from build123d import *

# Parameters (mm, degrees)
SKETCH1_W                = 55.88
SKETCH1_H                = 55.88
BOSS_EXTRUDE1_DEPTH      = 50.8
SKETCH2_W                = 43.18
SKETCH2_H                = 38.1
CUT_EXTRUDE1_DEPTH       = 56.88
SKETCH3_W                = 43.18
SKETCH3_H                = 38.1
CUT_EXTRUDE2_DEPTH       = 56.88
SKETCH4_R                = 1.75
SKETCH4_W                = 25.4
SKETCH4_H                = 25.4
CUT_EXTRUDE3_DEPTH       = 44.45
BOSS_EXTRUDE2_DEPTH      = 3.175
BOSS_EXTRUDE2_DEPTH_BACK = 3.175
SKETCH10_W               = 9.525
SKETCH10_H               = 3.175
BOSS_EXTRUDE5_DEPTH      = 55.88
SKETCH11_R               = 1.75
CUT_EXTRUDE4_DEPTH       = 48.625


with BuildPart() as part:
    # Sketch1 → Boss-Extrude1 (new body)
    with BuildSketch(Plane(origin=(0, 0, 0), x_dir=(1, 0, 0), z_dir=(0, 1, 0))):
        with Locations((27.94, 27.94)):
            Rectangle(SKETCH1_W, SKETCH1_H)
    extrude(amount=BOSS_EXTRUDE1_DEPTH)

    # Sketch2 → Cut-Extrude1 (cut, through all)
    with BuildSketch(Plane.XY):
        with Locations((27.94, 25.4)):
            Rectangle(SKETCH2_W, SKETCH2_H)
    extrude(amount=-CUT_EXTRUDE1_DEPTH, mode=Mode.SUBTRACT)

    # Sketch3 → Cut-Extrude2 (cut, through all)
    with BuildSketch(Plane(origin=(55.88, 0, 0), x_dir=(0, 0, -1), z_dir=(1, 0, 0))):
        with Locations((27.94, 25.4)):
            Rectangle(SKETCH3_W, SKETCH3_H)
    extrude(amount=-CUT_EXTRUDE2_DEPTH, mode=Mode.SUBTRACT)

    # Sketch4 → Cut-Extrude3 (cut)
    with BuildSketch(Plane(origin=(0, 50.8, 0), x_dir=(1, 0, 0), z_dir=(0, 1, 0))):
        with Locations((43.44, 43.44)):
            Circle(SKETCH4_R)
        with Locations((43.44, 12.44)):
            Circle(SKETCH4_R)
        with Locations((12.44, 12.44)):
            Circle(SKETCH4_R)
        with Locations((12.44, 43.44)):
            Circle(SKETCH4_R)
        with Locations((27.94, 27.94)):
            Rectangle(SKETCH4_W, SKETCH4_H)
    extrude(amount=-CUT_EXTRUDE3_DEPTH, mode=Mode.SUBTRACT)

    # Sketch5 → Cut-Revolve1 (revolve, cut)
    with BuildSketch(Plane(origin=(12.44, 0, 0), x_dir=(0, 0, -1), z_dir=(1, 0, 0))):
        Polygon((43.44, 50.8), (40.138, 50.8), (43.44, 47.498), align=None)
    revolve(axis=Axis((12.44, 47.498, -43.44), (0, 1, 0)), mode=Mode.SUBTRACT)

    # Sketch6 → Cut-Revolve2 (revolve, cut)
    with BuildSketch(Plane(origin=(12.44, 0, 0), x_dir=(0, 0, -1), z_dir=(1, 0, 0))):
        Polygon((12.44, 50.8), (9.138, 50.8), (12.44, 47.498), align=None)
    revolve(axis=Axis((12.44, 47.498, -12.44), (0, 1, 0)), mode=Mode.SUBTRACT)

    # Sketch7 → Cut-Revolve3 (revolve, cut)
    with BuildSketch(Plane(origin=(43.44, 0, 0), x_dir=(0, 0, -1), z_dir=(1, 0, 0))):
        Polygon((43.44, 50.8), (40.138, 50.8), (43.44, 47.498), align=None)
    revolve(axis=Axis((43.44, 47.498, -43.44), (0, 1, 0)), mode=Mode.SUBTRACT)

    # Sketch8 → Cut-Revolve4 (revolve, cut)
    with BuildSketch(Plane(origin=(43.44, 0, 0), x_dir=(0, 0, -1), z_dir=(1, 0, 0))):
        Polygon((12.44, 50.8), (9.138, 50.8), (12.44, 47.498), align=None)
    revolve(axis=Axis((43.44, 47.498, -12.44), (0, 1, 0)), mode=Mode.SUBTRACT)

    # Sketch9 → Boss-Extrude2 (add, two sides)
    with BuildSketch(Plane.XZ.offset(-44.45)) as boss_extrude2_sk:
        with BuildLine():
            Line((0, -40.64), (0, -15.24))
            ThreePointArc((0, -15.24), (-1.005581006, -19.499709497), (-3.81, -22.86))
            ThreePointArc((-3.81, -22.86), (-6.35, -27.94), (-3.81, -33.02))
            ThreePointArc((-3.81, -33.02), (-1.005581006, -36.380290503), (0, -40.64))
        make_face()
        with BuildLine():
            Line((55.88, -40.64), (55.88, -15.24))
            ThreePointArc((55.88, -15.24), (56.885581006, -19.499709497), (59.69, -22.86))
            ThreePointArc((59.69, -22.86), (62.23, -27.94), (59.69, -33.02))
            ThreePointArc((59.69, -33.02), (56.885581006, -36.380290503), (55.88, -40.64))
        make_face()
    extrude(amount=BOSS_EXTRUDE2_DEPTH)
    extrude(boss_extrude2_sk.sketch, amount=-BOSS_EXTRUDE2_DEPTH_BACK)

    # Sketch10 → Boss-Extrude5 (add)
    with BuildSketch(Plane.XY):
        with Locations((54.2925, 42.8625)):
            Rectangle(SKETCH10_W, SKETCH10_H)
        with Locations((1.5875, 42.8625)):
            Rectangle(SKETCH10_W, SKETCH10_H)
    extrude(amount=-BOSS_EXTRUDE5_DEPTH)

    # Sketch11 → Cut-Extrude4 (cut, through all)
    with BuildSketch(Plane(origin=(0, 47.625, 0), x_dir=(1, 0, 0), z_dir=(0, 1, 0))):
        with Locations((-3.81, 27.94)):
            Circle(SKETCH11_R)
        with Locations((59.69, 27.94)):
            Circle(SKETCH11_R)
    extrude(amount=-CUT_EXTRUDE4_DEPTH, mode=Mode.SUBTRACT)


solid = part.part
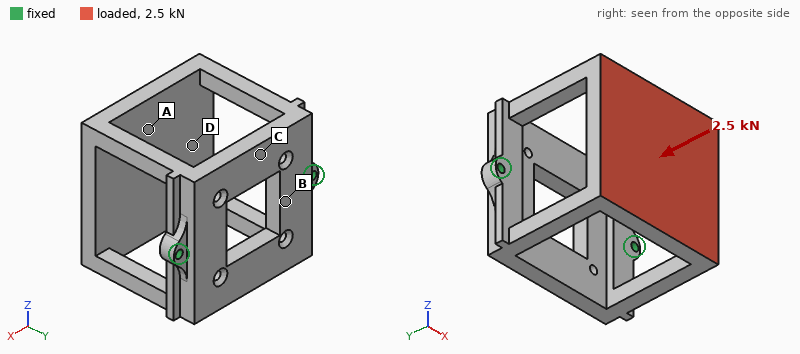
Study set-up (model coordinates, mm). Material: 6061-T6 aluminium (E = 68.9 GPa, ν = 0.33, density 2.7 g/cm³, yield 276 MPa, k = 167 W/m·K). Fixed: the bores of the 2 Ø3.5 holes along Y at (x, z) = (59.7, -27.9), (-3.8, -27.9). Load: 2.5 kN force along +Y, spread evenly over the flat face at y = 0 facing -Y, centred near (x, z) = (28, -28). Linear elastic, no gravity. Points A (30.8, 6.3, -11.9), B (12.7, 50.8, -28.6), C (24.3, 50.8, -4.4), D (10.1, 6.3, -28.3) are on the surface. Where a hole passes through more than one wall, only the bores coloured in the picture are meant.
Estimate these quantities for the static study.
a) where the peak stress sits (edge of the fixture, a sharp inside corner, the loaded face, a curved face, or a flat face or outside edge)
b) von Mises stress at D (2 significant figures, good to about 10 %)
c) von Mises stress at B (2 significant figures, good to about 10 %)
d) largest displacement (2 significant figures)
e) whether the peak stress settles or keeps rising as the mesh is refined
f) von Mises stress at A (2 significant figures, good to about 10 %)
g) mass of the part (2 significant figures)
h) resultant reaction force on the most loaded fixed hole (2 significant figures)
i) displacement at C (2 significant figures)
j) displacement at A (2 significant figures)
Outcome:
edge of the fixture
29 MPa
49 MPa
0.12 mm
keeps rising
24 MPa
120 g
1.4 kN
0.049 mm
0.11 mm
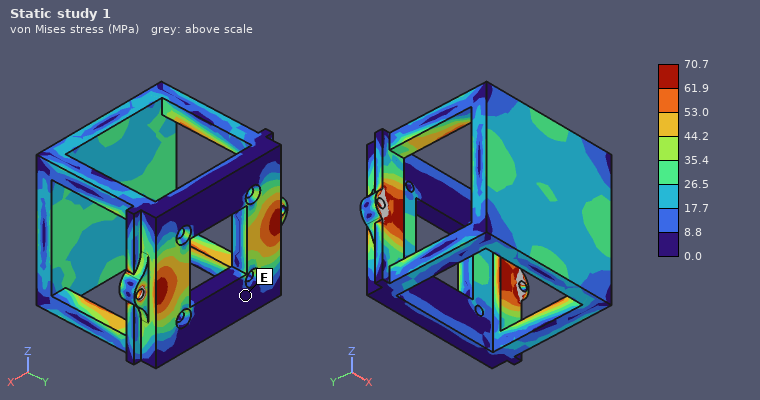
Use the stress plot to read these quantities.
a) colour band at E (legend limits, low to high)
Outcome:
0.0 to 8.8 MPa
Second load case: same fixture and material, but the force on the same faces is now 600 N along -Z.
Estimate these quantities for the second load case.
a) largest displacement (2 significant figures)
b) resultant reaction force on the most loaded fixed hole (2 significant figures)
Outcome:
0.35 mm
300 N
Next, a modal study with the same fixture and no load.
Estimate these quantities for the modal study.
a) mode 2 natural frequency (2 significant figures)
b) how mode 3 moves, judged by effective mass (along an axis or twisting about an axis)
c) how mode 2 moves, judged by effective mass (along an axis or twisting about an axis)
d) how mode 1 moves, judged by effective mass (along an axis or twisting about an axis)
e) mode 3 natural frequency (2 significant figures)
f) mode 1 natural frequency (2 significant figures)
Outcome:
1200 Hz
twisting about Y
along X
along Z
2100 Hz
880 Hz
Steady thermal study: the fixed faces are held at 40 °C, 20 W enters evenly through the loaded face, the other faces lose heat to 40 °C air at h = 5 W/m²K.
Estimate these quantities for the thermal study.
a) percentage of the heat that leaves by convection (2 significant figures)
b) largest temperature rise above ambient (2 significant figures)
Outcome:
7.6 %
40 K
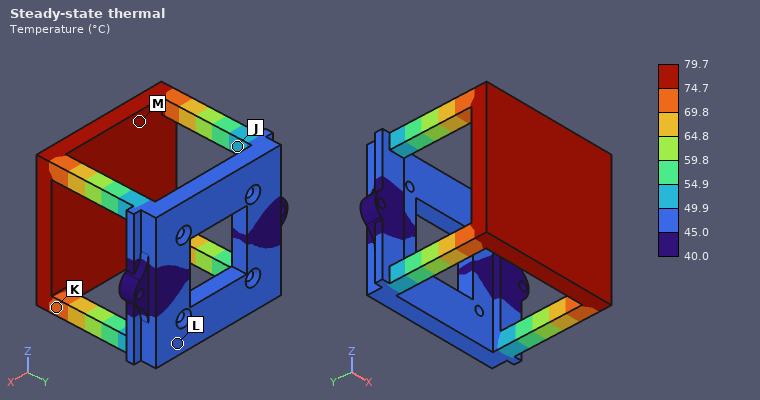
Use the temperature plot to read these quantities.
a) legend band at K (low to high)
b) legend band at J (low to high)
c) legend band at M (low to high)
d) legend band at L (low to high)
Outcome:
69.8 to 74.7 °C
49.9 to 54.9 °C
74.7 to 79.7 °C
45.0 to 49.9 °C
